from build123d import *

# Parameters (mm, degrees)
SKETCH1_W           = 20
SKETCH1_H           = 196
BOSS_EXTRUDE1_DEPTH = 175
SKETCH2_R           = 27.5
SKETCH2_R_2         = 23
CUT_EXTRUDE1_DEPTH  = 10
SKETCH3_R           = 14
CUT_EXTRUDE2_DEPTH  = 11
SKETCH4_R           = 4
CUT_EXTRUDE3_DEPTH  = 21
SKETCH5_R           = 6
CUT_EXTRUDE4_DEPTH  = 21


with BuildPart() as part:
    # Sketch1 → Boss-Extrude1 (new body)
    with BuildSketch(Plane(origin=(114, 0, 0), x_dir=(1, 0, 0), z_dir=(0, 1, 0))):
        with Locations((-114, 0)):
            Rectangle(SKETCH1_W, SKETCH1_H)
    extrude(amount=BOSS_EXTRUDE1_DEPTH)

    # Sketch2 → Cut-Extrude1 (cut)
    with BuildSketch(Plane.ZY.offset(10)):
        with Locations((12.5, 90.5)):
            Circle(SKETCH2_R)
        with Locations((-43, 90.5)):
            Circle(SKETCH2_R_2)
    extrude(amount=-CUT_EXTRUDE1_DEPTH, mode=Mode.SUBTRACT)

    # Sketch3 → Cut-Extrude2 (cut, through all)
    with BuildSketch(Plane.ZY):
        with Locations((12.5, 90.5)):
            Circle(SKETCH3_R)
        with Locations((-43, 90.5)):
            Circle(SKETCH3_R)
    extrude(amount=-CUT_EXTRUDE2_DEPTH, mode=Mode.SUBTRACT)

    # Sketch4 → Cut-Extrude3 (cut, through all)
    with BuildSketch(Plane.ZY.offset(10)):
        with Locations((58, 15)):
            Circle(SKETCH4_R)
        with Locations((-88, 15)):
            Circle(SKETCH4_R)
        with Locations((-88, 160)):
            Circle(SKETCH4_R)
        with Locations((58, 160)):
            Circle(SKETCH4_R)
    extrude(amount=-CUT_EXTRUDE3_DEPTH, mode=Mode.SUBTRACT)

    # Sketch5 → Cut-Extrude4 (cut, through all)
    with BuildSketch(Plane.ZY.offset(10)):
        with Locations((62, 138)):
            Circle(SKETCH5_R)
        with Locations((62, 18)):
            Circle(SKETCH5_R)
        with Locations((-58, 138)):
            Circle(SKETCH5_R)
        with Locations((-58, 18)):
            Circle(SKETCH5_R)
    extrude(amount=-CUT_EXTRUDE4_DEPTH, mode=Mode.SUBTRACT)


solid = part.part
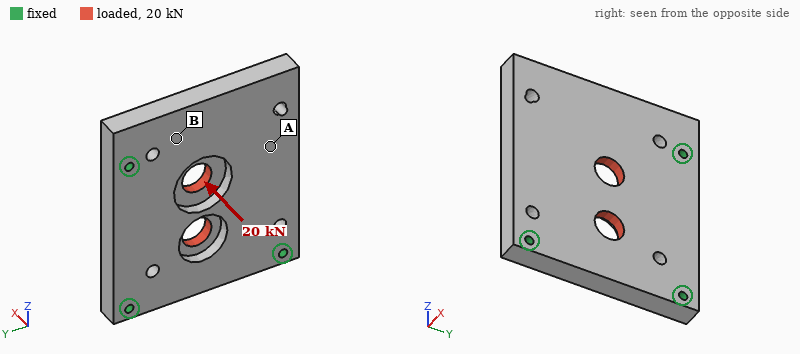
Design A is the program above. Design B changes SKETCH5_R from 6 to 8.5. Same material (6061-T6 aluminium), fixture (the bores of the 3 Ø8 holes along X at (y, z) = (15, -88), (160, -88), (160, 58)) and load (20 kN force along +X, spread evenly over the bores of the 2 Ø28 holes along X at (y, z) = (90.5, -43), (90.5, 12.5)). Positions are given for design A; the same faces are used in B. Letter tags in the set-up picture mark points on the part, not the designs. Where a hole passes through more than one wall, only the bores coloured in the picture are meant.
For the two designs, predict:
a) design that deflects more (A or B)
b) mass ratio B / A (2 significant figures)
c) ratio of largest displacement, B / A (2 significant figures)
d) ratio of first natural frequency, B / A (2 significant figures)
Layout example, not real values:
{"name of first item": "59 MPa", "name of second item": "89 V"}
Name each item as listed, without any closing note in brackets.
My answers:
{"design that deflects more": "B", "mass ratio B / A": "0.99", "ratio of largest displacement, B / A": "1.1", "ratio of first natural frequency, B / A": "0.98"}
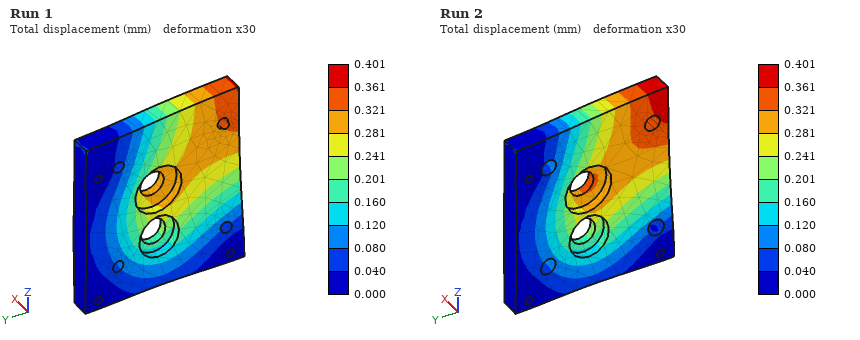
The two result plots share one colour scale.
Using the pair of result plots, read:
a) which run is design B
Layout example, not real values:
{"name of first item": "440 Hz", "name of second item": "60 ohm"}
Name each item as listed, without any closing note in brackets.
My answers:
{"which run is design B": "Run 2"}
